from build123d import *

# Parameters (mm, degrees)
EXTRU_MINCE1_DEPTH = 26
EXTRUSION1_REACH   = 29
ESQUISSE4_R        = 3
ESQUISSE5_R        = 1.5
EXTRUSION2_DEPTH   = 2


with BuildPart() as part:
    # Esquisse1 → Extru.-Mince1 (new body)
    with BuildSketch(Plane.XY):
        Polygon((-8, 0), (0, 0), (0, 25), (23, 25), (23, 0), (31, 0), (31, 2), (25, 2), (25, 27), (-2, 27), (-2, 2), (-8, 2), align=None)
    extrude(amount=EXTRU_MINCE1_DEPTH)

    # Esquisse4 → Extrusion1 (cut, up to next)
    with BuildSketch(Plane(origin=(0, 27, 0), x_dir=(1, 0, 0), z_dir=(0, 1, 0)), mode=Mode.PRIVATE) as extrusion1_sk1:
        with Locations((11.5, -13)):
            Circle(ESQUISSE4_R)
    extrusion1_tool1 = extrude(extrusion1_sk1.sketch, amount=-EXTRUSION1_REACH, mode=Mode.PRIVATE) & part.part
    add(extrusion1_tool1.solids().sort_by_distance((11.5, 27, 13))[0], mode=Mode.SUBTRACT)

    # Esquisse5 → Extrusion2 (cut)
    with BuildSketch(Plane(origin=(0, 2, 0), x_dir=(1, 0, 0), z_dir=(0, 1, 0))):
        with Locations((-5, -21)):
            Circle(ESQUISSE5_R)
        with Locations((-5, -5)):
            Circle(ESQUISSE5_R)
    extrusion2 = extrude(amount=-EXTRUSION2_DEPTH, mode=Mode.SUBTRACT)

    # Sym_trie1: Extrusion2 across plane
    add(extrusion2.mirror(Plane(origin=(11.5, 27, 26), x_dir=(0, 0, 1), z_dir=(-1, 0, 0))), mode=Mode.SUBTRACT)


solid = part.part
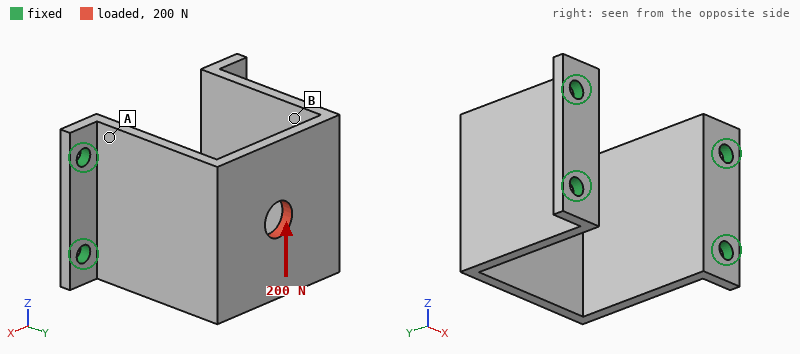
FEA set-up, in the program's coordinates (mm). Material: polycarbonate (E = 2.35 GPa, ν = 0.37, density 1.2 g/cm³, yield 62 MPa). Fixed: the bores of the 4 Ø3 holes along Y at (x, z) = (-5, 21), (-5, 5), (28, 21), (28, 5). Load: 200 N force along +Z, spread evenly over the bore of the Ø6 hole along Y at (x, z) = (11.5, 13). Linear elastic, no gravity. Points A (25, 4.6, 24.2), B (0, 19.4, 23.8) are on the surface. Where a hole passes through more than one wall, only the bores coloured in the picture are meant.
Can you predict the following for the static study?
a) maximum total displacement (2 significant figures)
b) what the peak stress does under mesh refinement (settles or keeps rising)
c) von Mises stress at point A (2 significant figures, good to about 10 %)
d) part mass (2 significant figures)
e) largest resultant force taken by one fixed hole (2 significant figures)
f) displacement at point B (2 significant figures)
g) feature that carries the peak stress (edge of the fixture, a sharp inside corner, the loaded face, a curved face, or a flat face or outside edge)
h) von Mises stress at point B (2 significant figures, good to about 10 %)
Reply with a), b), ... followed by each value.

a) 0.53 mm
b) keeps rising
c) 19 MPa
d) 5.4 g
e) 150 N
f) 0.37 mm
g) edge of the fixture
h) 5.1 MPa
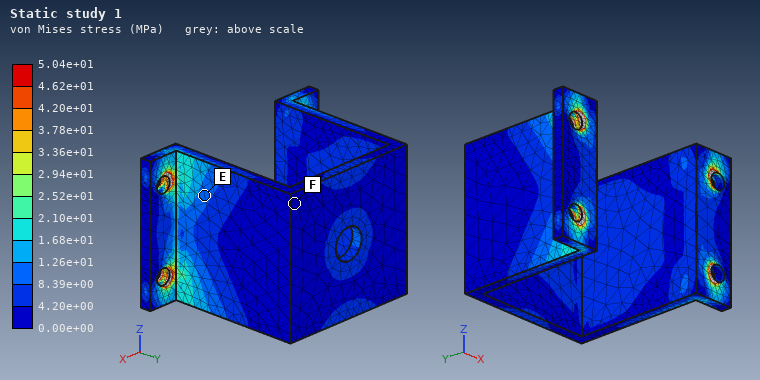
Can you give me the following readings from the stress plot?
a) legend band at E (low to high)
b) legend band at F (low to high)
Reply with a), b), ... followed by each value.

a) 8.39e+00 to 1.26e+01 MPa
b) 0.00e+00 to 4.20e+00 MPa
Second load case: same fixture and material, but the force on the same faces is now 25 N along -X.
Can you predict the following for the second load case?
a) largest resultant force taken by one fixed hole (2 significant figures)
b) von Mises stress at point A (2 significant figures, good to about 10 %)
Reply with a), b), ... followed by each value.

a) 9.0 N
b) 6.2 MPa
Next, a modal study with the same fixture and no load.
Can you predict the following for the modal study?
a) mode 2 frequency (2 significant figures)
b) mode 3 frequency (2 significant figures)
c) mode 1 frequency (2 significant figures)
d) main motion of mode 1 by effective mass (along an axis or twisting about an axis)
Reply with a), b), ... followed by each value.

a) 1900 Hz
b) 2000 Hz
c) 630 Hz
d) along X
